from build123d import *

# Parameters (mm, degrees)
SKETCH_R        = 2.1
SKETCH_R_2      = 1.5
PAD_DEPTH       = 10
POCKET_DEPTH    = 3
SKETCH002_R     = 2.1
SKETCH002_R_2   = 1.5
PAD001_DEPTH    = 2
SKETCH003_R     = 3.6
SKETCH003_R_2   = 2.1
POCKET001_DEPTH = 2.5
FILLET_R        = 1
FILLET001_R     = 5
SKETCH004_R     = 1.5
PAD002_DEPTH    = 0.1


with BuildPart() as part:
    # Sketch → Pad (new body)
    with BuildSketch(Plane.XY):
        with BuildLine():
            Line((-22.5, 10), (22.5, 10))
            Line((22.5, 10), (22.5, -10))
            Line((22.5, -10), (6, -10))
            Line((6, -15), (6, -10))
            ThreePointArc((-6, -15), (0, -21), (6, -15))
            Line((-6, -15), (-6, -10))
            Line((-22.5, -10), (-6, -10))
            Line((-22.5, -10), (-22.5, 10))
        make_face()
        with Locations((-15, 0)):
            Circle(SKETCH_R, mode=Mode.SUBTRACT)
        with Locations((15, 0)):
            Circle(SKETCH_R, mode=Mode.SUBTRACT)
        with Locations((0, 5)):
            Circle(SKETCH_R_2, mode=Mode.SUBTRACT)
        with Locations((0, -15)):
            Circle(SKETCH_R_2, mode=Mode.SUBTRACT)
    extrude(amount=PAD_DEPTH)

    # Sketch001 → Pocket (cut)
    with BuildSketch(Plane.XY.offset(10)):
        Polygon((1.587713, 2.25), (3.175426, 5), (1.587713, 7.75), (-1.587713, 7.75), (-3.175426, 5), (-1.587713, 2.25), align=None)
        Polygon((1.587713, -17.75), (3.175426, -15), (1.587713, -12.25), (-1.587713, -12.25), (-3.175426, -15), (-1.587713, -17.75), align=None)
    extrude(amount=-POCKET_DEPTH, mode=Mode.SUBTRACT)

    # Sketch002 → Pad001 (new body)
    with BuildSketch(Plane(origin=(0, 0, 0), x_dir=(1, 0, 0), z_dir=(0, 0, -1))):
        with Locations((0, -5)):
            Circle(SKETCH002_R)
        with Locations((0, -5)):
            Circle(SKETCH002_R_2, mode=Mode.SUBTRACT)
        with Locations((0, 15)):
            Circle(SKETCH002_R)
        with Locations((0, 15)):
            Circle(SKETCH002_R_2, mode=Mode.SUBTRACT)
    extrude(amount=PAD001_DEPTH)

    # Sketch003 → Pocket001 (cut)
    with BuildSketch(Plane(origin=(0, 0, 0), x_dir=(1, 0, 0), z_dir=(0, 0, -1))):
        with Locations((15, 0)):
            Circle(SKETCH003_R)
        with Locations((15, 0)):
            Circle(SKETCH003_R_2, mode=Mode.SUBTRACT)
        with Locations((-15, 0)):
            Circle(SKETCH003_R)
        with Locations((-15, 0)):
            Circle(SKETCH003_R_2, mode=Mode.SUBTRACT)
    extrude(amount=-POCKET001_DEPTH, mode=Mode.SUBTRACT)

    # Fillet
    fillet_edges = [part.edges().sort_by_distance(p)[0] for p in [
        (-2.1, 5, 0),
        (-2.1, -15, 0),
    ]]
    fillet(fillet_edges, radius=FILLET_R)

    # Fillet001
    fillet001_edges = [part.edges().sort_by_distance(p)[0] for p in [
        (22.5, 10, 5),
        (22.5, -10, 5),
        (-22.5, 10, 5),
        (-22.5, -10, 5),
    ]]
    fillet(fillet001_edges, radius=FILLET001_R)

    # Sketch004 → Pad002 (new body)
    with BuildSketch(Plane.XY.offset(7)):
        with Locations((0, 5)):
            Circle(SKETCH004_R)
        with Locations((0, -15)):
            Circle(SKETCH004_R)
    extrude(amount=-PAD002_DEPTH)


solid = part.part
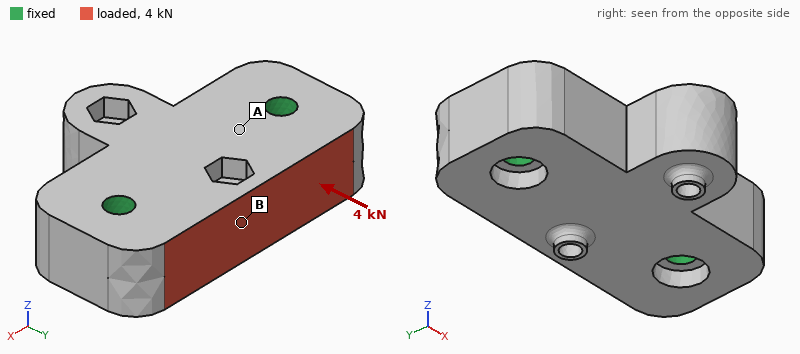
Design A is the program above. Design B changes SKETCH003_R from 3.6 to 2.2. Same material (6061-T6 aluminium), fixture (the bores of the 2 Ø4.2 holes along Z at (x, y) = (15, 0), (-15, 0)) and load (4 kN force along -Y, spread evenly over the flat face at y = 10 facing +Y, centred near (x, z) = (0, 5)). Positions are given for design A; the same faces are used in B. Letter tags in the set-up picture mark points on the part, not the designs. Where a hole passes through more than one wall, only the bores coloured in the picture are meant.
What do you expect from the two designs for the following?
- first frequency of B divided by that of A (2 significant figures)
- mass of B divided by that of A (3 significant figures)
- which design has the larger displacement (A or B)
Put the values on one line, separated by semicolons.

1.0; 1.01; A
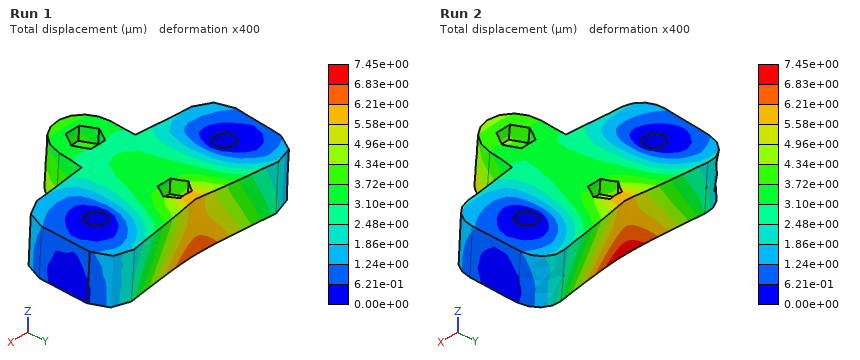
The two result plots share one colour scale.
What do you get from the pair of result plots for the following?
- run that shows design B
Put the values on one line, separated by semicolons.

Run 1
